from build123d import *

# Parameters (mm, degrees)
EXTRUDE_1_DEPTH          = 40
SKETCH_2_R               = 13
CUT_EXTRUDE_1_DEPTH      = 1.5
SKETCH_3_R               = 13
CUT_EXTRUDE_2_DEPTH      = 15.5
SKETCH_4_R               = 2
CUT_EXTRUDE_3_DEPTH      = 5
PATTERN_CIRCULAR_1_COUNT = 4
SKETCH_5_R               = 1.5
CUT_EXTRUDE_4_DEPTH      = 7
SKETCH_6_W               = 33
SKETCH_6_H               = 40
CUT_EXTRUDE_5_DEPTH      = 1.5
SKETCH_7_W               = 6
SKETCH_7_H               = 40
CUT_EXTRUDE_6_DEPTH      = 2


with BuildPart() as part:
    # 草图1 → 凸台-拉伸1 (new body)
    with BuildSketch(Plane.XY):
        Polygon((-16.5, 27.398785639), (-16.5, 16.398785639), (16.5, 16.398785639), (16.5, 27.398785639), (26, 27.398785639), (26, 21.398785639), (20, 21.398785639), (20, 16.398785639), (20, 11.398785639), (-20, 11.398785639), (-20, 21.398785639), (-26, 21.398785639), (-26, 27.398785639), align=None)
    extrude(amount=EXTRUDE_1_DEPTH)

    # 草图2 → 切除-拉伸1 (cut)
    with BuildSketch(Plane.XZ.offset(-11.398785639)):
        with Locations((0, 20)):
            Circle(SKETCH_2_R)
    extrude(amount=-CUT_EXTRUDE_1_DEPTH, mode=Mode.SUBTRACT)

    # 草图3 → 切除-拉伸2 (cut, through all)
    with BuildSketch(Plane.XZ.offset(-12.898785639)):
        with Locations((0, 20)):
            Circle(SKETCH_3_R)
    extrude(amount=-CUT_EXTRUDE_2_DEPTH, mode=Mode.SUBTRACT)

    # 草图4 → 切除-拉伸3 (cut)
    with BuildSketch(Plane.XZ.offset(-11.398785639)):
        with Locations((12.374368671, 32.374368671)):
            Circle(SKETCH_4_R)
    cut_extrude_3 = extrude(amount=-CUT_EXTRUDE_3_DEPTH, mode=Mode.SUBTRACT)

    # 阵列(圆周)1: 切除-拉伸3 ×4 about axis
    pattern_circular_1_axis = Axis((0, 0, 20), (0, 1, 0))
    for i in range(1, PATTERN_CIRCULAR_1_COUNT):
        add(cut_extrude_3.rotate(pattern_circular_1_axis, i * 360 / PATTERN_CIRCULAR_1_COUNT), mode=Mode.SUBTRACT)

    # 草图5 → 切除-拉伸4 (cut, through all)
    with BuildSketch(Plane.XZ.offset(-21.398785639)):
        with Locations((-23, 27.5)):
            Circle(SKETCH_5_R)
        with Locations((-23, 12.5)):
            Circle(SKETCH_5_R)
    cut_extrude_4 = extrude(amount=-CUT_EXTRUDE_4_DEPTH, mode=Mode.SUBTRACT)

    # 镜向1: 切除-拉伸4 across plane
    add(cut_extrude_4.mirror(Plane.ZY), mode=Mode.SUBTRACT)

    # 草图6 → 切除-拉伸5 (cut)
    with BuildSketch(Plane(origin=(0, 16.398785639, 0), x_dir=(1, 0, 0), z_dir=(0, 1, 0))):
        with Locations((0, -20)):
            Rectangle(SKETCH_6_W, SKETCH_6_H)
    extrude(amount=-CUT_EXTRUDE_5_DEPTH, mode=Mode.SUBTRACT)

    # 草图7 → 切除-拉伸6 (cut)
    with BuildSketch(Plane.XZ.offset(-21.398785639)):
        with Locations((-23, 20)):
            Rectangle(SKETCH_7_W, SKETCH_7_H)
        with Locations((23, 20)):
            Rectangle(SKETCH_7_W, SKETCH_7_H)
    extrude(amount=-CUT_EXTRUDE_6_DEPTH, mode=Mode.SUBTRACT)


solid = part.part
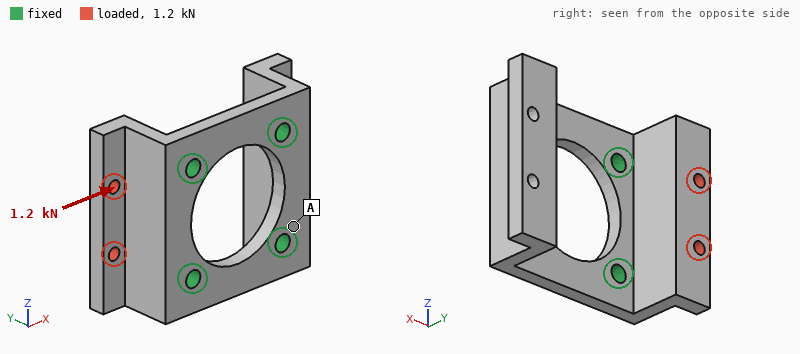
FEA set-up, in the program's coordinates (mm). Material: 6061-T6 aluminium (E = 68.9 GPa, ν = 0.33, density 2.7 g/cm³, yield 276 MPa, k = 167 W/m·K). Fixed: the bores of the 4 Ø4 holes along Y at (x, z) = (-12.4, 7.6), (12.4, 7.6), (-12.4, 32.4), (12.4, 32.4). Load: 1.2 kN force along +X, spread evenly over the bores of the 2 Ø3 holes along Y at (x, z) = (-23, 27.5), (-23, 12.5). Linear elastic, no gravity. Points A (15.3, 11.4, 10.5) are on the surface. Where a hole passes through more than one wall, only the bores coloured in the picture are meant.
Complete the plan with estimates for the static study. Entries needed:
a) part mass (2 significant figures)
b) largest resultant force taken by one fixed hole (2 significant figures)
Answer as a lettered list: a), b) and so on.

a) 24 g
b) 630 N
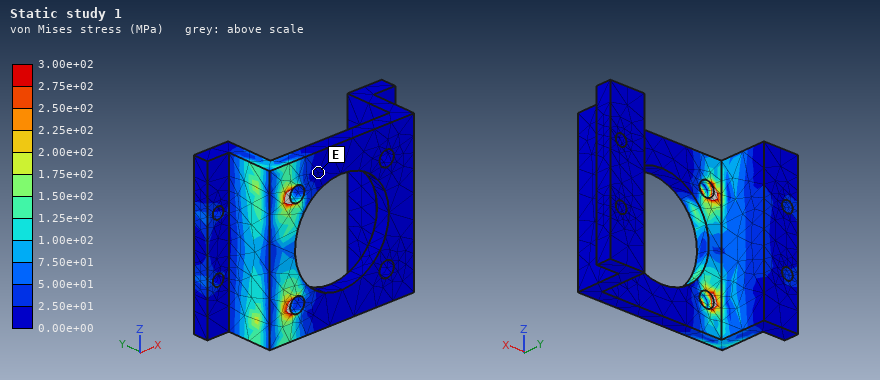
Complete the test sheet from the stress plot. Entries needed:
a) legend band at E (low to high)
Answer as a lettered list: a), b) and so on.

a) 0.00e+00 to 2.50e+01 MPa
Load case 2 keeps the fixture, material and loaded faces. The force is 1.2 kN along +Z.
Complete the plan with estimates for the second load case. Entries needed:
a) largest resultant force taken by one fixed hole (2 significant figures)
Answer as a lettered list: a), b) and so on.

a) 890 N
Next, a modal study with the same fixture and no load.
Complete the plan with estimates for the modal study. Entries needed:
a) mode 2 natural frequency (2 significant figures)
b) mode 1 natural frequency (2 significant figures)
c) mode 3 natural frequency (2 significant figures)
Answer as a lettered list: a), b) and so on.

a) 5400 Hz
b) 5400 Hz
c) 9900 Hz
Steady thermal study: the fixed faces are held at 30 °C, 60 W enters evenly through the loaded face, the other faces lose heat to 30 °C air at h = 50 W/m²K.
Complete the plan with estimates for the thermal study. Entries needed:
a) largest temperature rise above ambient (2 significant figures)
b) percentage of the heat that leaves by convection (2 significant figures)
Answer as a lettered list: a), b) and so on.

a) 66 K
b) 6.6 %
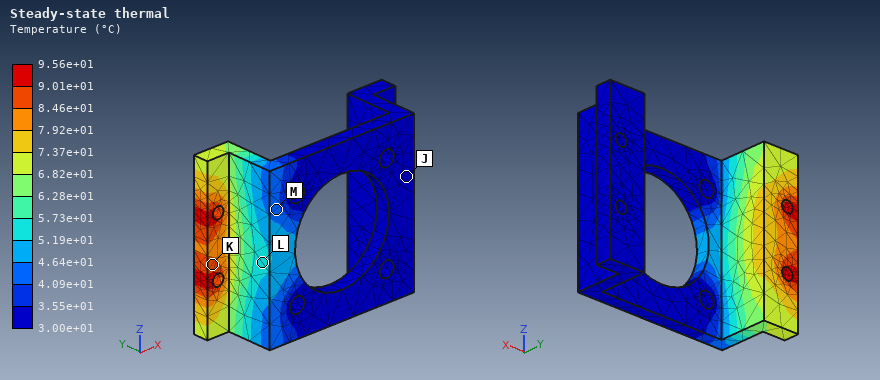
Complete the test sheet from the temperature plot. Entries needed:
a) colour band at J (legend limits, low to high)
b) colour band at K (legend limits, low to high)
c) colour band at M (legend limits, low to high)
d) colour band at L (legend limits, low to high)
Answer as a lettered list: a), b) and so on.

a) 3.00e+01 to 3.55e+01 °C
b) 8.46e+01 to 9.01e+01 °C
c) 4.09e+01 to 4.64e+01 °C
d) 5.19e+01 to 5.73e+01 °C
